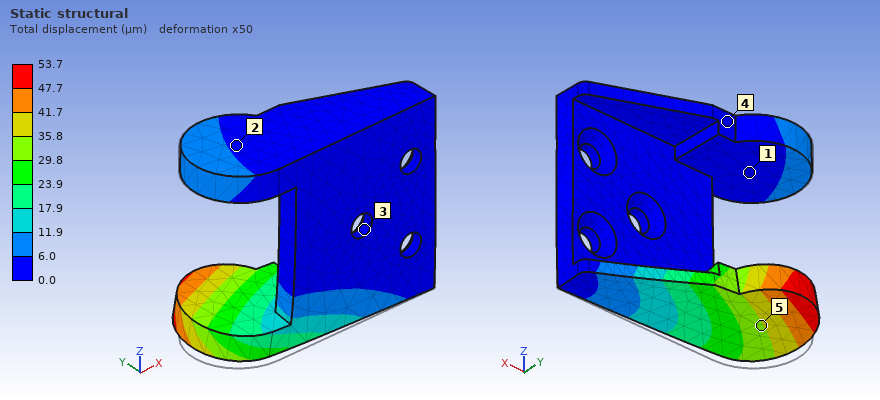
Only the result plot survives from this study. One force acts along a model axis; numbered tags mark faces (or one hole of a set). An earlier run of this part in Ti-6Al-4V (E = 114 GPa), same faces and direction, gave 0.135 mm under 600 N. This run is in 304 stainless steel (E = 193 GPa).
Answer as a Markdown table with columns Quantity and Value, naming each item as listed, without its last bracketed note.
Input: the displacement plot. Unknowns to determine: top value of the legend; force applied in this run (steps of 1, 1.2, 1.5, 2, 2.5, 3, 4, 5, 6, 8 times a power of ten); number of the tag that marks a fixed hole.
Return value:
| Quantity | Value |
|---|---|
| top value of the legend | 53.7 µm |
| force applied in this run | 400 N |
| number of the tag that marks a fixed hole | 3 |
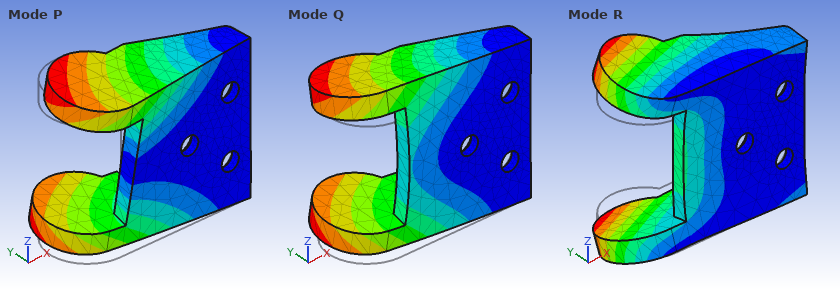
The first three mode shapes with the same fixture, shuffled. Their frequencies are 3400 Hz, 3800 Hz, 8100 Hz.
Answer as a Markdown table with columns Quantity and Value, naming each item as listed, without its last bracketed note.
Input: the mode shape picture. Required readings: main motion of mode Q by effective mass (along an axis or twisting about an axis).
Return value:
| Quantity | Value |
|---|---|
| main motion of mode Q by effective mass | along Y |
